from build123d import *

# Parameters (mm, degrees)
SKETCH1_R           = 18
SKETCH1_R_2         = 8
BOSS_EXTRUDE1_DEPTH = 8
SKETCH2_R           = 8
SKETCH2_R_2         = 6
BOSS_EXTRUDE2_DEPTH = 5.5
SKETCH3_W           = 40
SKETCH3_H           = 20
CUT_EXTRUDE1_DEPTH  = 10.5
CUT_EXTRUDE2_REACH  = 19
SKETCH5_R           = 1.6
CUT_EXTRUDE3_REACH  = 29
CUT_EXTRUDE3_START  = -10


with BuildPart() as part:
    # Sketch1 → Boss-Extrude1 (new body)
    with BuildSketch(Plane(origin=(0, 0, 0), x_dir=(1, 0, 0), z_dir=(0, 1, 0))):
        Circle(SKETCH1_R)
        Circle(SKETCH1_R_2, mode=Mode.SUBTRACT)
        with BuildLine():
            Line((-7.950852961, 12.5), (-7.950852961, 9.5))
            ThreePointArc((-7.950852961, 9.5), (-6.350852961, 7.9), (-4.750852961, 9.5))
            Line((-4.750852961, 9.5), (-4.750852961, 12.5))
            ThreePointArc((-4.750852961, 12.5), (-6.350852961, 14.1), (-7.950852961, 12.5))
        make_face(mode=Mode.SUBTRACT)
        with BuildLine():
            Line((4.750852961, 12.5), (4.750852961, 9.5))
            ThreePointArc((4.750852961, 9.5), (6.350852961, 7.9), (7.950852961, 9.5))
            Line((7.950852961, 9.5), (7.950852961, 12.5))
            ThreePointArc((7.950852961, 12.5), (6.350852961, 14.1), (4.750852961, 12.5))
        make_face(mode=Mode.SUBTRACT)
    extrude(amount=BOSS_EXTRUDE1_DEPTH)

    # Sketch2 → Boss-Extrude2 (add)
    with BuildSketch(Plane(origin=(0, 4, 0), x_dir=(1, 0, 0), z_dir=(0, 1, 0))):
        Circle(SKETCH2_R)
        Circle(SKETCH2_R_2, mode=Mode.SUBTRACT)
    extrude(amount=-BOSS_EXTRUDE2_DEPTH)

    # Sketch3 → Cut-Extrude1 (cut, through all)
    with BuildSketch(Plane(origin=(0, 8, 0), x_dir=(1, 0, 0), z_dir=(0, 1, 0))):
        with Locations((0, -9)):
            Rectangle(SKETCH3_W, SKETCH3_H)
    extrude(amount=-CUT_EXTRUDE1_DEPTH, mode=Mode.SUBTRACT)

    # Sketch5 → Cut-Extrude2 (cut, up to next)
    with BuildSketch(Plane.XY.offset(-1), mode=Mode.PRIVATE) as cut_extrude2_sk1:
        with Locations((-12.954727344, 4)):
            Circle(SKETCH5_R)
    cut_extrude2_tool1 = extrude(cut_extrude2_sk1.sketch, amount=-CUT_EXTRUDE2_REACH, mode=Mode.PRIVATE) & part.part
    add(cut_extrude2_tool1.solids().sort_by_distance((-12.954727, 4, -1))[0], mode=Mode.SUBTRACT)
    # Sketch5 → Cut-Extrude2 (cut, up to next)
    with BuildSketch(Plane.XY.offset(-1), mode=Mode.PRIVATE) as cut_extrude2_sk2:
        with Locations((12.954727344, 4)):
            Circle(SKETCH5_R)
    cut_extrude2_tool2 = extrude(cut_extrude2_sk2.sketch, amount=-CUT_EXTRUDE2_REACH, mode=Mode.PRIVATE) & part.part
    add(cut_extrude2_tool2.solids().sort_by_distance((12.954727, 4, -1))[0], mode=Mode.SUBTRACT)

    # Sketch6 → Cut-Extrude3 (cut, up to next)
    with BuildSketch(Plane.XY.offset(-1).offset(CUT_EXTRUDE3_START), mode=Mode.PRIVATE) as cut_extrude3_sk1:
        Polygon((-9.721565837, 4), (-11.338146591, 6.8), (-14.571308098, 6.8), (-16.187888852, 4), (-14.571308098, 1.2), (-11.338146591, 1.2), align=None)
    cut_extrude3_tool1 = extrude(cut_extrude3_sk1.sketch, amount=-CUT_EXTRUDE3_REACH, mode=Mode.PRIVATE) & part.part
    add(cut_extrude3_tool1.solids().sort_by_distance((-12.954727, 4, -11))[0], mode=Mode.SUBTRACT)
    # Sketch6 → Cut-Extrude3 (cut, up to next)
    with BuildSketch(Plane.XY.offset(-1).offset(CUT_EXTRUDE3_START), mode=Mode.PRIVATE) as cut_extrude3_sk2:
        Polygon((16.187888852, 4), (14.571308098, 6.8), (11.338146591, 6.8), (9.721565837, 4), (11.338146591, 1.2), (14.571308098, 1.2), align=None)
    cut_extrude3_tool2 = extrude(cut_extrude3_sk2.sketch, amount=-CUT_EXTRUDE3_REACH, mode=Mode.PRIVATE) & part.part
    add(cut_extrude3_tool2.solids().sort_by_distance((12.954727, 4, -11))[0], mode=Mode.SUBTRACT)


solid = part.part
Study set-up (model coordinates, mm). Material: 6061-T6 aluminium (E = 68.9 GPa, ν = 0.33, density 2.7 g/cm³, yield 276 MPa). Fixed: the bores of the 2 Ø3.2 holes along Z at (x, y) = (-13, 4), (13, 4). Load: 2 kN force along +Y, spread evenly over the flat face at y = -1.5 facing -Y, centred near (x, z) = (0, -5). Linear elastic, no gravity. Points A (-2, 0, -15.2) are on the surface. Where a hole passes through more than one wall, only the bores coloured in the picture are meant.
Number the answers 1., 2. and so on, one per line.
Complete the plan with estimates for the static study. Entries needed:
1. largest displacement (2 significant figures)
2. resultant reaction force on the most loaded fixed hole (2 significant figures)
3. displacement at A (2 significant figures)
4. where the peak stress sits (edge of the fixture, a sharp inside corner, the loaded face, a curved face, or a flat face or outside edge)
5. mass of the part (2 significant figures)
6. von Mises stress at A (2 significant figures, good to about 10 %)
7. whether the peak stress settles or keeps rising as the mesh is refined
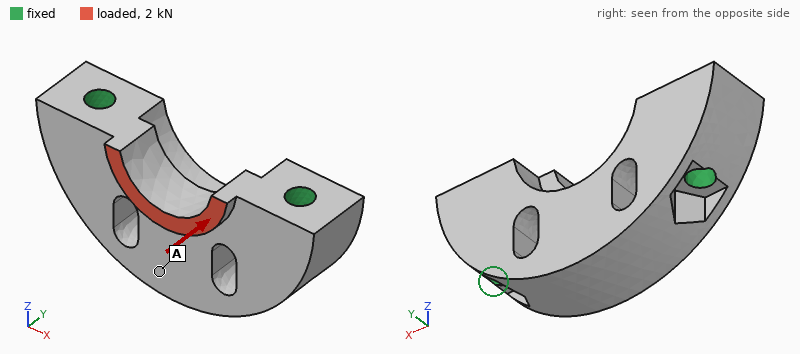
1. 17 µm
2. 1.0 kN
3. 6.4 µm
4. edge of the fixture
5. 7.6 g
6. 17 MPa
7. keeps rising
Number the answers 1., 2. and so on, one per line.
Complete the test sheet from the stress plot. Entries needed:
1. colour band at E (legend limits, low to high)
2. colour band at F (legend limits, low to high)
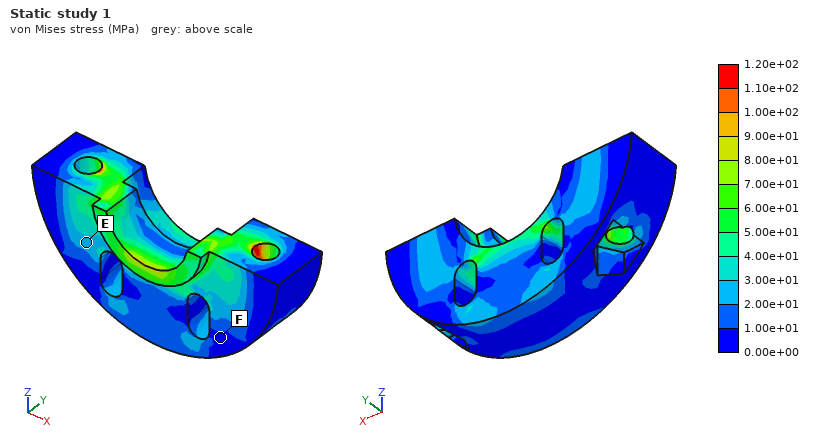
1. 2.00e+01 to 3.00e+01 MPa
2. 0.00e+00 to 1.00e+01 MPa
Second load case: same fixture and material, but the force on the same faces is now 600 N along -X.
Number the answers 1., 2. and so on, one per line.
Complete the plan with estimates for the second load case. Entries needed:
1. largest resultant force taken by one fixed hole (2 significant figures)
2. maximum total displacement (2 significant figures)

1. 320 N
2. 5.6 µm
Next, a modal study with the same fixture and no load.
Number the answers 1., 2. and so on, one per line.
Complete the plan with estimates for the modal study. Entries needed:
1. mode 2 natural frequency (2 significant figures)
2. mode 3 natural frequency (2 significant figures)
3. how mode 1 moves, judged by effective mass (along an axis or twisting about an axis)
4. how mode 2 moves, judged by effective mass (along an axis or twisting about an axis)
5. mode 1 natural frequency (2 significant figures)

1. 44 kHz
2. 52 kHz
3. along Y
4. along Z
5. 25 kHz
